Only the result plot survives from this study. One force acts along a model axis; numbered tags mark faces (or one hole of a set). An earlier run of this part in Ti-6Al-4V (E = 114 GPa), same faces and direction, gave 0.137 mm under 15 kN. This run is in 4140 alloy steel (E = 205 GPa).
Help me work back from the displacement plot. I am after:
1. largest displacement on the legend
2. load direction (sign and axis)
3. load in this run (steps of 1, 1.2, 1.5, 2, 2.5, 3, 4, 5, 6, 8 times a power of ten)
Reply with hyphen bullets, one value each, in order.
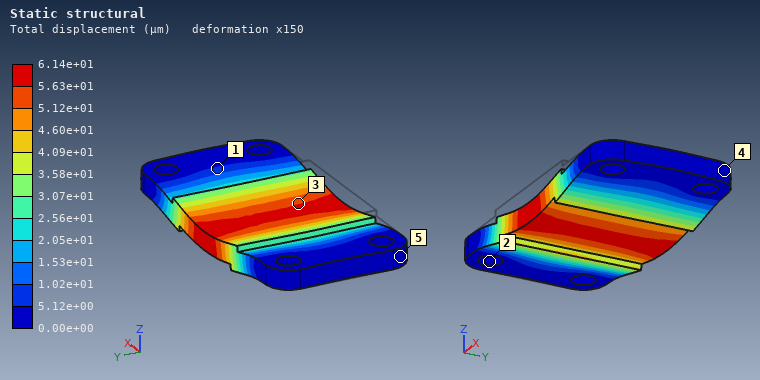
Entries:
- 6.14e+01 µm
- -Z
- 12 kN
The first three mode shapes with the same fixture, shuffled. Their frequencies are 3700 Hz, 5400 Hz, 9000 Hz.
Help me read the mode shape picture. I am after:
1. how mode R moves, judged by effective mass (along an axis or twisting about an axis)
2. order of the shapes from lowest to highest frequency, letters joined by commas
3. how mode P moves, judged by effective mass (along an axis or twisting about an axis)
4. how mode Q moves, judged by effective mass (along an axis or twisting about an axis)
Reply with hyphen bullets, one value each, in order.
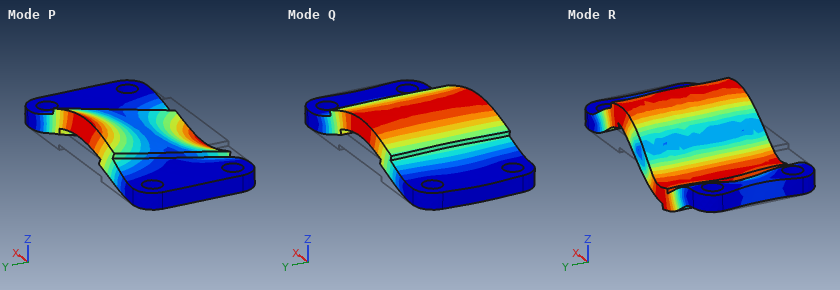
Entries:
- twisting about Y
- Q, P, R
- twisting about X
- along Z
